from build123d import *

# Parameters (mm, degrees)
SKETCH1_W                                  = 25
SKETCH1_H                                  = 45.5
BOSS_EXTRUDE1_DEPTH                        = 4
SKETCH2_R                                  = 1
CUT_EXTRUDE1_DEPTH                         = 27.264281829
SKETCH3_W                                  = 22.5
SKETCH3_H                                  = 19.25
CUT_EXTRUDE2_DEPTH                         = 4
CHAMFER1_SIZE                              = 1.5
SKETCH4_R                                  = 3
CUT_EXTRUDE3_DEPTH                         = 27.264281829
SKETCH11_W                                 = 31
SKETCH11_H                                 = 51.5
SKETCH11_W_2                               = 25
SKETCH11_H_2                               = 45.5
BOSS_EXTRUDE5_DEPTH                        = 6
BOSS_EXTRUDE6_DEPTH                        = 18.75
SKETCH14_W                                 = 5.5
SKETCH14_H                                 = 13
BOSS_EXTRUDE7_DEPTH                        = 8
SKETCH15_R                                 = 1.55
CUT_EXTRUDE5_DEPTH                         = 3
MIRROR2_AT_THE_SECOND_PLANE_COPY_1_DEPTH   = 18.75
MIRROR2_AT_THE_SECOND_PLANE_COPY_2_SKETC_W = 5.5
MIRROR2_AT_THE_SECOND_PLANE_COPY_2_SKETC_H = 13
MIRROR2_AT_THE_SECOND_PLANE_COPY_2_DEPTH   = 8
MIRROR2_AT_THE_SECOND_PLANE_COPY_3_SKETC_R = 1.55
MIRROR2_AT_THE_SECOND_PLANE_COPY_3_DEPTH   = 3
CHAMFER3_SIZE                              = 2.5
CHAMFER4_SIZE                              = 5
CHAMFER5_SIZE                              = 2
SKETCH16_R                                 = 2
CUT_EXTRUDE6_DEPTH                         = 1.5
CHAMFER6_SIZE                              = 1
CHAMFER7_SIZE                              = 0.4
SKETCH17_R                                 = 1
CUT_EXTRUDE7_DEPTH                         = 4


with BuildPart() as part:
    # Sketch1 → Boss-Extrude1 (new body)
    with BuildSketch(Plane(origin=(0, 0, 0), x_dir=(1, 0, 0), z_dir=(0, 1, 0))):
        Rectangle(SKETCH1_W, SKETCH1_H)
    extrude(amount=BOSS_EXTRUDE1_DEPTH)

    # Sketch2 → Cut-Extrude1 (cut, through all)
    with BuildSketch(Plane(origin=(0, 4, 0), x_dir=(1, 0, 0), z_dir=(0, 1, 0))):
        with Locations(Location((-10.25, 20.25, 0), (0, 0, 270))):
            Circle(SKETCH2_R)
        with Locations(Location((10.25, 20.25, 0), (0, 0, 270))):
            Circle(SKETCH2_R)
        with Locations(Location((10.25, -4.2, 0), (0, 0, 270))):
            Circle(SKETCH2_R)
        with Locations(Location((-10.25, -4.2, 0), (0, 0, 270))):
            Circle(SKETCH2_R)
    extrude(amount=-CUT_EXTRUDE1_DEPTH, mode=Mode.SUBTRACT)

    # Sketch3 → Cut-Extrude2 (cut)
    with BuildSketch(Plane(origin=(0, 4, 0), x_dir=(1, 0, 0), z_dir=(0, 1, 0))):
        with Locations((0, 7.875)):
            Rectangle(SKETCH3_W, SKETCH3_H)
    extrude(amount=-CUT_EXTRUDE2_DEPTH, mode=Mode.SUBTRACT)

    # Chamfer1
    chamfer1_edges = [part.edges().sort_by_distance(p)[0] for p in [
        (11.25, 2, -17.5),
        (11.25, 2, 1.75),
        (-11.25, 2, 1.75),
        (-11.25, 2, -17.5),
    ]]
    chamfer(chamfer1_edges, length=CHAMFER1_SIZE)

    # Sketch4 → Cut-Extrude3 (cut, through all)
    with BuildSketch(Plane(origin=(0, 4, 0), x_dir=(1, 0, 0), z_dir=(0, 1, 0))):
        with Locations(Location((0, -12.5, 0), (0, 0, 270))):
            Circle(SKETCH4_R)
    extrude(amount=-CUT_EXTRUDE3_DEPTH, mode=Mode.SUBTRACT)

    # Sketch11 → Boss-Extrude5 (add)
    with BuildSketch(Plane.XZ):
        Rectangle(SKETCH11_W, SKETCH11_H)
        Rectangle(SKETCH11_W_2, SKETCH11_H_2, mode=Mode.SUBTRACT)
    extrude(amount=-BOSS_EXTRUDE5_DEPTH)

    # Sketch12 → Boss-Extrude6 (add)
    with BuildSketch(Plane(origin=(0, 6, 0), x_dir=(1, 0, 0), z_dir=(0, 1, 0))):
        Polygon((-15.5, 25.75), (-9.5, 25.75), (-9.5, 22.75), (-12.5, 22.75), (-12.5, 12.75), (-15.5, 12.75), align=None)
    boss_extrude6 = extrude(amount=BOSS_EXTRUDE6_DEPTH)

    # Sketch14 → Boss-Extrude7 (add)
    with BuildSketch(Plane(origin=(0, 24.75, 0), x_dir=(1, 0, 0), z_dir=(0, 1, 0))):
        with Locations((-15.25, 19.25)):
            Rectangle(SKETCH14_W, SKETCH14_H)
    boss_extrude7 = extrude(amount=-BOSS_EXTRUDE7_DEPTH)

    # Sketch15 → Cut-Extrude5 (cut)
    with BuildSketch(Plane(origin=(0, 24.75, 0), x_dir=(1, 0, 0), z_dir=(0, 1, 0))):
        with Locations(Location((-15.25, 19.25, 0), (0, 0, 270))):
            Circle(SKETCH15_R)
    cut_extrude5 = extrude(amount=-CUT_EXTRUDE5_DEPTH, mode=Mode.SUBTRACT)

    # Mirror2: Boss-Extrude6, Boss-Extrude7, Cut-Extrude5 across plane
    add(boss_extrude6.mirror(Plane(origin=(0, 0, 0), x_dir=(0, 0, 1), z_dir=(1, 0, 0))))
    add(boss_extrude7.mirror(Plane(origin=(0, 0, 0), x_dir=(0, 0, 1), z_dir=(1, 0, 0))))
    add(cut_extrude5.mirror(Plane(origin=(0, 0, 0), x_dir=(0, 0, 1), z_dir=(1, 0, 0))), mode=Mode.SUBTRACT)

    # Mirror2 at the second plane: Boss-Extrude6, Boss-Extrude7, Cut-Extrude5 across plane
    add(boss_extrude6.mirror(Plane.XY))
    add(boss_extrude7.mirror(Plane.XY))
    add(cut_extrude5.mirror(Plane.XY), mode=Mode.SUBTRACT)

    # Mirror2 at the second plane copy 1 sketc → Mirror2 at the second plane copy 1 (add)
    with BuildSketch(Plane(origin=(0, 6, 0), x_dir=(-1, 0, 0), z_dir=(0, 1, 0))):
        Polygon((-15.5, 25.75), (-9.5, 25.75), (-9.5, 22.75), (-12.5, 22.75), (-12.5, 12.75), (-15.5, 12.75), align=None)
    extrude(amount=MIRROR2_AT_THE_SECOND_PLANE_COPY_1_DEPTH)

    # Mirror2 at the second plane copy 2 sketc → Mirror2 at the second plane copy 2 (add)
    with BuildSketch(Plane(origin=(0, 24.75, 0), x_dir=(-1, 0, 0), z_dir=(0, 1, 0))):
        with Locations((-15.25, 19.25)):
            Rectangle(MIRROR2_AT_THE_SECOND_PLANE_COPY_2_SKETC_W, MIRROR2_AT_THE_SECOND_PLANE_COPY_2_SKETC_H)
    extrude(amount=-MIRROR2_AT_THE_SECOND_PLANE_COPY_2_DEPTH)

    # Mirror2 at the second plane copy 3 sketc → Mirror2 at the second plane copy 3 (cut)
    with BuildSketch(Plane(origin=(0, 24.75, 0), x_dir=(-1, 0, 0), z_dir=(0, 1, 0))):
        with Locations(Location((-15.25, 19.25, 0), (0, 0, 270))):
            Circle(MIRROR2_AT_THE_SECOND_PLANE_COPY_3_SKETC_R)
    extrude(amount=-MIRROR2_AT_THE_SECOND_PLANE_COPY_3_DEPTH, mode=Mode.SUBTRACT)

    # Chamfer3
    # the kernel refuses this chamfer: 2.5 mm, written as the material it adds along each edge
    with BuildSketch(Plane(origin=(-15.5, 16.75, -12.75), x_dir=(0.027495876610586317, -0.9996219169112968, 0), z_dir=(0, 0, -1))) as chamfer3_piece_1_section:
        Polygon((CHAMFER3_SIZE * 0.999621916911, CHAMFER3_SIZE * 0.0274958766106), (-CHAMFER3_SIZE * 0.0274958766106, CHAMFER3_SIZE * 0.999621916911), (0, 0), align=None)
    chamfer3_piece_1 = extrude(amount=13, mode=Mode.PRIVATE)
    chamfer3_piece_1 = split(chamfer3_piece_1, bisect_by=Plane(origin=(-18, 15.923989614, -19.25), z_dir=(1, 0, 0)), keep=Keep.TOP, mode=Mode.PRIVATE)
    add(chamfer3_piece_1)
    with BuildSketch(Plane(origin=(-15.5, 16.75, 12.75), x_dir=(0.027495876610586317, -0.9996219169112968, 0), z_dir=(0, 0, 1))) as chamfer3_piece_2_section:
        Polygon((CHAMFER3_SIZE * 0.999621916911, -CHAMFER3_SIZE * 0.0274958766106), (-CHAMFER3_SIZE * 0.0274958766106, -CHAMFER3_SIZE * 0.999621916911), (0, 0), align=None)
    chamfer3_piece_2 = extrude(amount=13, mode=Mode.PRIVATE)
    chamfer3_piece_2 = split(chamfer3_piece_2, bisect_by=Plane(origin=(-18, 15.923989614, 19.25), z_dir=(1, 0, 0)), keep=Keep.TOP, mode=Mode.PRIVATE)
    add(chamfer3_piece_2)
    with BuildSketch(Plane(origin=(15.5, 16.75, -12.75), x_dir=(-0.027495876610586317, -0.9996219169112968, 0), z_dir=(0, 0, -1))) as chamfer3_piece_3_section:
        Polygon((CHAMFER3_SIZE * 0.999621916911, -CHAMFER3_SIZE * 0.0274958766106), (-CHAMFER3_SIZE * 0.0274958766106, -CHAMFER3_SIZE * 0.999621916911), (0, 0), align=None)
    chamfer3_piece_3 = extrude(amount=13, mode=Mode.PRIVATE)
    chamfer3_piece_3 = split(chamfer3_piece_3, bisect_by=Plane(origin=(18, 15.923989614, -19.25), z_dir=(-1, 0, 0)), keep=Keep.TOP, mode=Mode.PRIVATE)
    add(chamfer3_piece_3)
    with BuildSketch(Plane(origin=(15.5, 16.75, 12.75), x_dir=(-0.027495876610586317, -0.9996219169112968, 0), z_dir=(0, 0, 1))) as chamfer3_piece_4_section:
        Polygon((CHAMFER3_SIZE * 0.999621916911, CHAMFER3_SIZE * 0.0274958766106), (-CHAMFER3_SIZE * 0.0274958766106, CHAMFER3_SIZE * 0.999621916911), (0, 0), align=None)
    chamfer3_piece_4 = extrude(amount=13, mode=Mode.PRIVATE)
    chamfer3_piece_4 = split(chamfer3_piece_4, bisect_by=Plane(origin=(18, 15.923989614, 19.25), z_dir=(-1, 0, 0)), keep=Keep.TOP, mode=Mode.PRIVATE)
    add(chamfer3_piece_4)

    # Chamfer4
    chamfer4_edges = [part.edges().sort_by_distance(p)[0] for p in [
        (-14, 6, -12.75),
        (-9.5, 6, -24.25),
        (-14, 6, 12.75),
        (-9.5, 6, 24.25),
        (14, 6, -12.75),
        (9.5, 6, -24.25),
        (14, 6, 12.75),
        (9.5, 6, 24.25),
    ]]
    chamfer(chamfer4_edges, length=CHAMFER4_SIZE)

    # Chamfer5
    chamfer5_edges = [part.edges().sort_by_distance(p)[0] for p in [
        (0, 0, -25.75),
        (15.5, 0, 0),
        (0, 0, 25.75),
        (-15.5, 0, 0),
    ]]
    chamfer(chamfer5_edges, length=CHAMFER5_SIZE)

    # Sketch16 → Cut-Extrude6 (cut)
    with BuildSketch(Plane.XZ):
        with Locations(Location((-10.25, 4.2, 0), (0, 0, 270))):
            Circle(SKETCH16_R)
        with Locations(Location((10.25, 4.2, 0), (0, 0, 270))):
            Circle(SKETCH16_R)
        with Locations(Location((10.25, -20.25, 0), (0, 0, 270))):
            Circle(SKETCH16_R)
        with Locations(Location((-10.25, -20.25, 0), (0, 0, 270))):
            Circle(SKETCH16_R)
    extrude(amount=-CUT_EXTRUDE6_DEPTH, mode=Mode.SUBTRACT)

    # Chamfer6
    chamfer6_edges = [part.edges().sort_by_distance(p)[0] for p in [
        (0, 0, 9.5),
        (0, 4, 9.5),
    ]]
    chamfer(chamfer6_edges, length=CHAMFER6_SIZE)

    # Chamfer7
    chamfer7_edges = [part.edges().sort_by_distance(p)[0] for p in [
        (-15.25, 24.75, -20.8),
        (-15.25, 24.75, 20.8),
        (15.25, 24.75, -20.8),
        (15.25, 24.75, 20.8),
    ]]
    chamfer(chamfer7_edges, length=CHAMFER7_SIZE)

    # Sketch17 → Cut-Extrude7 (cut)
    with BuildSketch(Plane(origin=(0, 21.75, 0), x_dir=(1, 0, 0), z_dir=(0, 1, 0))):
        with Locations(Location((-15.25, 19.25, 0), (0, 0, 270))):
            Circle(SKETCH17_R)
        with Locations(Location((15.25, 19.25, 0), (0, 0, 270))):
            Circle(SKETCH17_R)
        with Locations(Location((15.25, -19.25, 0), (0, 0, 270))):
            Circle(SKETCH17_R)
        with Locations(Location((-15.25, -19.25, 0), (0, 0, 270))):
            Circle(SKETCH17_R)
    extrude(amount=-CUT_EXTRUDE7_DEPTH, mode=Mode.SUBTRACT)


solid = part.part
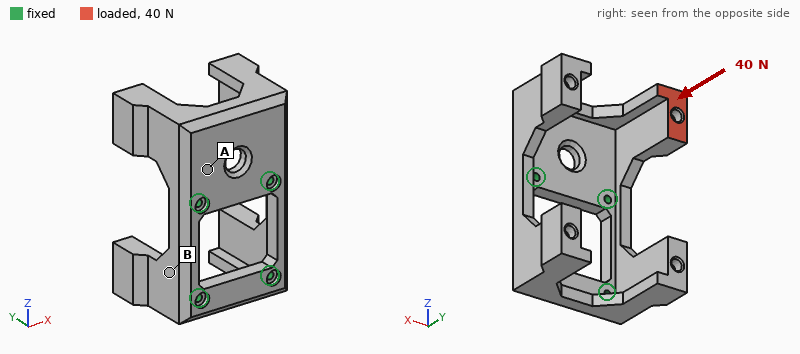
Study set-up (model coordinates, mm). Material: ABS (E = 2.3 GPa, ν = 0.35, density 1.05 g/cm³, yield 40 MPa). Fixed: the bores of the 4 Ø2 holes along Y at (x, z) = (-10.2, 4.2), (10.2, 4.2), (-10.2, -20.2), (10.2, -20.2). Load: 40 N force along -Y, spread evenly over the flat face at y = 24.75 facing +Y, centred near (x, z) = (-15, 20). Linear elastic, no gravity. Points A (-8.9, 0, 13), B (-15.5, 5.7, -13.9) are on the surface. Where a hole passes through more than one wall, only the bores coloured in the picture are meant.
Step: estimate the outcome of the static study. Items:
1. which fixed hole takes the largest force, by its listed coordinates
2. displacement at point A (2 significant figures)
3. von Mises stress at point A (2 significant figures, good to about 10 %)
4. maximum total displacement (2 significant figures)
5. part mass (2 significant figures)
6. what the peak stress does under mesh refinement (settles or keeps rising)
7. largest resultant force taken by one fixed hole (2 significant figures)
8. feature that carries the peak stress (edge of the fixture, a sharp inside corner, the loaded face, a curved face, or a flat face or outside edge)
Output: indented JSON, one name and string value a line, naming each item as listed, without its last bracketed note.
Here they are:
{
  "which fixed hole takes the largest force, by its listed coordinates": "(-10.2, 4.2)",
  "displacement at point A": "0.16 mm",
  "von Mises stress at point A": "4.3 MPa",
  "maximum total displacement": "0.80 mm",
  "part mass": "10 g",
  "what the peak stress does under mesh refinement": "keeps rising",
  "largest resultant force taken by one fixed hole": "54 N",
  "feature that carries the peak stress": "edge of the fixture"
}
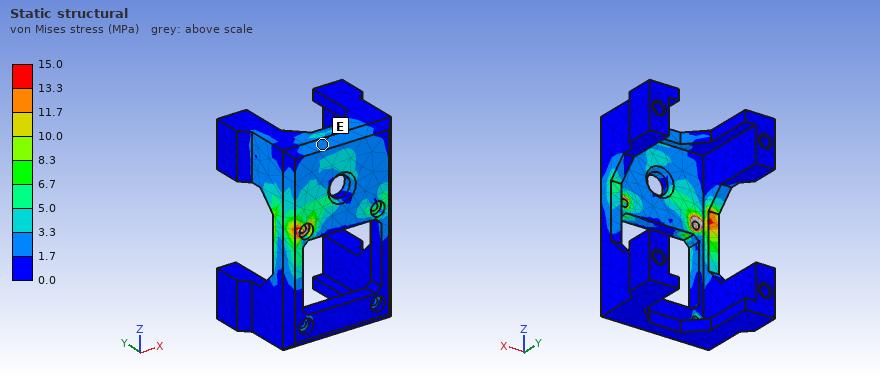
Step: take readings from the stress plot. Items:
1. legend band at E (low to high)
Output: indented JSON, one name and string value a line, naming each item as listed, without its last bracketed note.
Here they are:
{
  "legend band at E": "1.7 to 3.3 MPa"
}
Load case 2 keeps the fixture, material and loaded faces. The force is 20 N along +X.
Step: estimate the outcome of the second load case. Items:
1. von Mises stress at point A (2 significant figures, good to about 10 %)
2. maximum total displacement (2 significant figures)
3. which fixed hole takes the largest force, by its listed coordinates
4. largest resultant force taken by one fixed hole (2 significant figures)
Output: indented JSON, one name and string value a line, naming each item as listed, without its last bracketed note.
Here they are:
{
  "von Mises stress at point A": "4.1 MPa",
  "maximum total displacement": "0.65 mm",
  "which fixed hole takes the largest force, by its listed coordinates": "(-10.2, 4.2)",
  "largest resultant force taken by one fixed hole": "30 N"
}
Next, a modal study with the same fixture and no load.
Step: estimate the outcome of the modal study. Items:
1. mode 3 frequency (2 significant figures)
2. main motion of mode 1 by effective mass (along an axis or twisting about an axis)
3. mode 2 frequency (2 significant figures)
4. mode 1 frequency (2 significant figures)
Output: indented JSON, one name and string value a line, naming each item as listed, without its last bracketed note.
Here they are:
{
  "mode 3 frequency": "1400 Hz",
  "main motion of mode 1 by effective mass": "along Y",
  "mode 2 frequency": "920 Hz",
  "mode 1 frequency": "770 Hz"
}
